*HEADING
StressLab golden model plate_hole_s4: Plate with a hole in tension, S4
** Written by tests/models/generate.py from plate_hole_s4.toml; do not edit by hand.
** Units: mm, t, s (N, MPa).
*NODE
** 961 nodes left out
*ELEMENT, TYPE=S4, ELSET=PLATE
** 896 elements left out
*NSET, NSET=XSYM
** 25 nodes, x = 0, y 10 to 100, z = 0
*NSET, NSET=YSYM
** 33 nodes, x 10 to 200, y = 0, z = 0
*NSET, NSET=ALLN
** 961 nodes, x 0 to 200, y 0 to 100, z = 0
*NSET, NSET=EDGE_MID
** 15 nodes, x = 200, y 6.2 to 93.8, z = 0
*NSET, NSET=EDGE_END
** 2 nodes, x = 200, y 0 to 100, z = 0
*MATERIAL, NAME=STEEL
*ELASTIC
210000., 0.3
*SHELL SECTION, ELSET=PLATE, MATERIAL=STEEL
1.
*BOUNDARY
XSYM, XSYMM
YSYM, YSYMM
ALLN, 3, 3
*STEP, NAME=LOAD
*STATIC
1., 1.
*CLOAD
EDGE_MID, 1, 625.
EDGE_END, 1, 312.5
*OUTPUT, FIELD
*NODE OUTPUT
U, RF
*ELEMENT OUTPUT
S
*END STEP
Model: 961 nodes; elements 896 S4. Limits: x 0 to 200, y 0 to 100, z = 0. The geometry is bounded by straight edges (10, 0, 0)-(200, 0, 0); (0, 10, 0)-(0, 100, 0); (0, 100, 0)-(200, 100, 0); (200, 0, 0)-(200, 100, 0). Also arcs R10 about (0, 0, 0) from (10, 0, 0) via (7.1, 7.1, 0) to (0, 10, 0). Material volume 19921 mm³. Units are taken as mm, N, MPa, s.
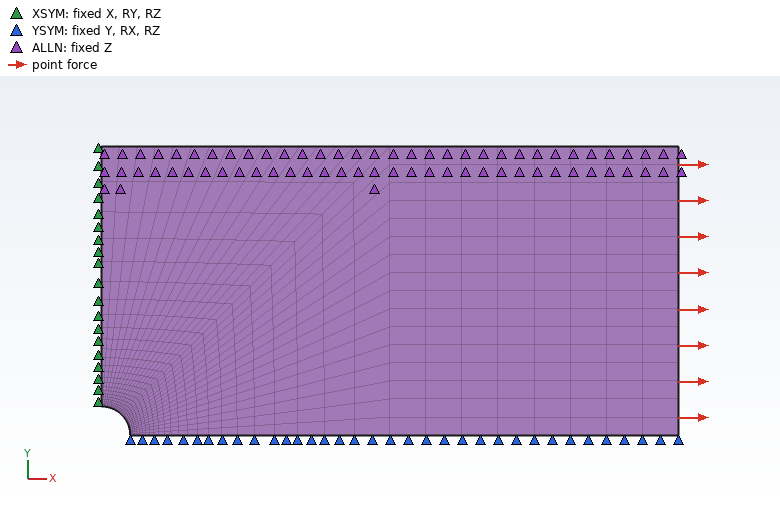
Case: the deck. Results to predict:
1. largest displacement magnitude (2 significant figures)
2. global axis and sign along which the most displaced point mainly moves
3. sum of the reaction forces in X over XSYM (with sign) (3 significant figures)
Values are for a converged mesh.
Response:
0.10 mm
+X
-10000 N
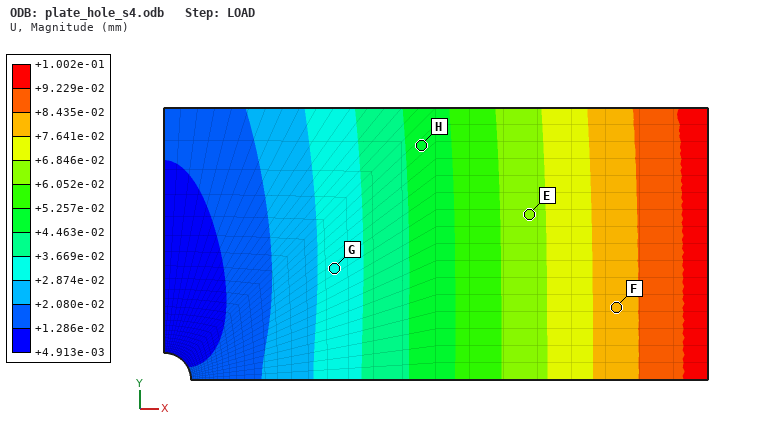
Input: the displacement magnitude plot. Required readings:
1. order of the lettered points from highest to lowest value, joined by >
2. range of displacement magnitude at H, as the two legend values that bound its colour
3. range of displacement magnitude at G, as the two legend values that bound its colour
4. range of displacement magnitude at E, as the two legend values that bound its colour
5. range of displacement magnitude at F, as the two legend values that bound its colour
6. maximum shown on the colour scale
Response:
F > E > H > G
+4.463e-02 to +5.257e-02 mm
+2.874e-02 to +3.669e-02 mm
+6.052e-02 to +6.846e-02 mm
+7.641e-02 to +8.435e-02 mm
+1.002e-01 mm
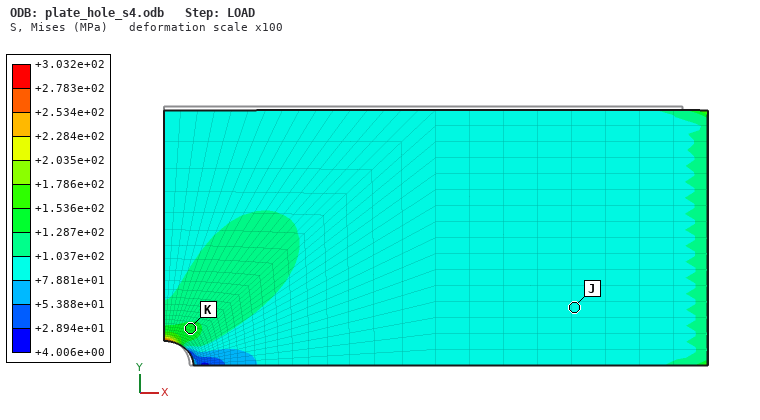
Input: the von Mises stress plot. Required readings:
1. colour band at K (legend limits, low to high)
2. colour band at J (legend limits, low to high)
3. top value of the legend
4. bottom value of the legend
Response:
+1.287e+02 to +1.536e+02 MPa
+7.881e+01 to +1.037e+02 MPa
+3.032e+02 MPa
+4.006e+00 MPa
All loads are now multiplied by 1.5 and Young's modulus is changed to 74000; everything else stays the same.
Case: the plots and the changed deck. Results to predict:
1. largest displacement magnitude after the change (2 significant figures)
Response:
0.43 mm
